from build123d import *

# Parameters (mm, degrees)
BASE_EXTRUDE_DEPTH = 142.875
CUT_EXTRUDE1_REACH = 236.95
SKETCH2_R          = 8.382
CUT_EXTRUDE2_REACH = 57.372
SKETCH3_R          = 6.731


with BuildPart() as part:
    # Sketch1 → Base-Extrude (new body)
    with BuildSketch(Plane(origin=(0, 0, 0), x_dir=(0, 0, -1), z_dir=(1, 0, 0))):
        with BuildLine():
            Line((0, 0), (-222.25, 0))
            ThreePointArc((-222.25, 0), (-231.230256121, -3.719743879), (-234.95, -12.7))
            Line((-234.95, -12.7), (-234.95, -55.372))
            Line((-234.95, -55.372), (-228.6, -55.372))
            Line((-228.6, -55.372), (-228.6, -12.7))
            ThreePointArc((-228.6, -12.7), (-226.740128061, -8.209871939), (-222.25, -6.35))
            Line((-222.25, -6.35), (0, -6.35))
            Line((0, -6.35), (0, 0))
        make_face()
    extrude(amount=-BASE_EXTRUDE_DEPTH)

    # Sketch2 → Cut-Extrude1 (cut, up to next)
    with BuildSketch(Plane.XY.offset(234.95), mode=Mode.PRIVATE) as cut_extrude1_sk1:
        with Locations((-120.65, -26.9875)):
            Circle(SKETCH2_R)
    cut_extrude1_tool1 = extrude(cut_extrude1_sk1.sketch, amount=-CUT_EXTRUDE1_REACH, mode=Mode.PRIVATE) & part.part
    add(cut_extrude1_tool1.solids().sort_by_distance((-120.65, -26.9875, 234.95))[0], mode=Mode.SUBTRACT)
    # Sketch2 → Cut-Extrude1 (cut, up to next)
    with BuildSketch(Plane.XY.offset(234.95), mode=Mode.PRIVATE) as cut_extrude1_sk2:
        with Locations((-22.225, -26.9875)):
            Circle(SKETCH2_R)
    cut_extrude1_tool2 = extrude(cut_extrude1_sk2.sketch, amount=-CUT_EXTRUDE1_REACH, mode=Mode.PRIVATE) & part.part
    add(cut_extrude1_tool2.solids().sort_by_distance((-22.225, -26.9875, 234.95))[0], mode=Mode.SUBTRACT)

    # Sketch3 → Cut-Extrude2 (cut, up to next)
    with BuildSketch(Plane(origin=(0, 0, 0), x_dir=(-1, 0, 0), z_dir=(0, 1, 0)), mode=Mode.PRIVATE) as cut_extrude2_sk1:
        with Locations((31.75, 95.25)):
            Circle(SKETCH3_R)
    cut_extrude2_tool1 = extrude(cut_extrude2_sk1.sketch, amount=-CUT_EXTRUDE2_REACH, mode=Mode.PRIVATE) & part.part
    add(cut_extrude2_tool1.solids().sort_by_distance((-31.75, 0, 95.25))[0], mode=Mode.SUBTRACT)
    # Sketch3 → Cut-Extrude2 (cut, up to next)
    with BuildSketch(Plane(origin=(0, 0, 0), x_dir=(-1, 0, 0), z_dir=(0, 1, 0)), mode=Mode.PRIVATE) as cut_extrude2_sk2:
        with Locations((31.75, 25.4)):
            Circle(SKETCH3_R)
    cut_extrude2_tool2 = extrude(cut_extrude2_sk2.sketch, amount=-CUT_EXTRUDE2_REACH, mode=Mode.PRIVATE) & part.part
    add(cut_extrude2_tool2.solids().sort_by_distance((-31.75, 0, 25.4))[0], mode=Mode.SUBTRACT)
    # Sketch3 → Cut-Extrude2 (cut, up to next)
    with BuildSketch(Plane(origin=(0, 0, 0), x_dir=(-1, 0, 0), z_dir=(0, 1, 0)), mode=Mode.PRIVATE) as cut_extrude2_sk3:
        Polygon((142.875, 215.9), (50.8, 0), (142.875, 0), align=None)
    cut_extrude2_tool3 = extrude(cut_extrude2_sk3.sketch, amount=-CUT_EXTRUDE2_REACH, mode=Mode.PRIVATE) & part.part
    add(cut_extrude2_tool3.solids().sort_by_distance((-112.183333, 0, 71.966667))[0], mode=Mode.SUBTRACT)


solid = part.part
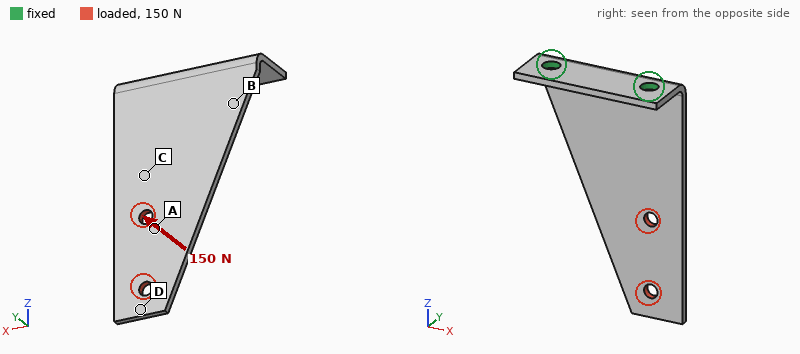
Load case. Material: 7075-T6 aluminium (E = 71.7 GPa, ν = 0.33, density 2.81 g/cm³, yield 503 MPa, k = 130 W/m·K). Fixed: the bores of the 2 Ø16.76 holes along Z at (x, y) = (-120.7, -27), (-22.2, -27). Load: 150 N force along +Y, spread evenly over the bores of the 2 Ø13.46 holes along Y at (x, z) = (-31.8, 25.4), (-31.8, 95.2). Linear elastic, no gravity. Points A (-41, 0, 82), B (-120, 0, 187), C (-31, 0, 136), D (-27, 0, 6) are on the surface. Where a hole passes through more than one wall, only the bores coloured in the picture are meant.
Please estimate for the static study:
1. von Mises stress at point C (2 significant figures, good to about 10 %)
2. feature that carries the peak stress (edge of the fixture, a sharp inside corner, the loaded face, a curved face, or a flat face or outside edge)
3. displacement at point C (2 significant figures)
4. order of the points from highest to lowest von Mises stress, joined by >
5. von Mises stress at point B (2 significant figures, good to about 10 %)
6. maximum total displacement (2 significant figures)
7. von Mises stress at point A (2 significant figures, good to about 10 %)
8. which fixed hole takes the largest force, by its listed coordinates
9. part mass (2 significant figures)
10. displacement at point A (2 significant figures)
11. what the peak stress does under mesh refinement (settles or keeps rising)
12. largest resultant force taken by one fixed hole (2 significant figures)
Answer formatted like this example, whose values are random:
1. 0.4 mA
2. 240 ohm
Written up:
1. 16 MPa
2. edge of the fixture
3. 0.69 mm
4. B > C > A > D
5. 22 MPa
6. 2.6 mm
7. 8.9 MPa
8. (-22.2, -27)
9. 520 g
10. 1.3 mm
11. keeps rising
12. 130 N
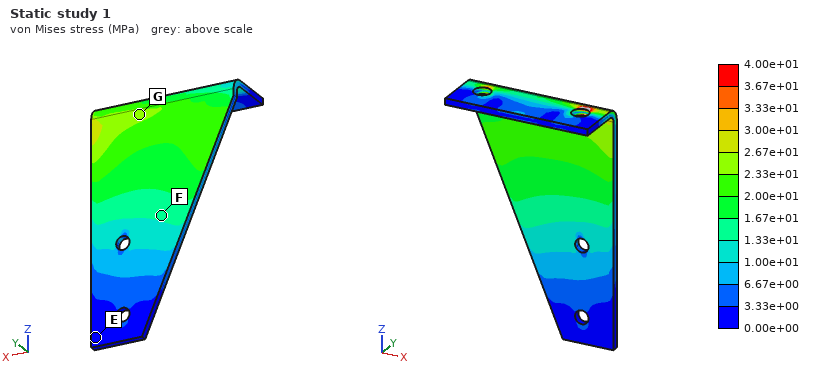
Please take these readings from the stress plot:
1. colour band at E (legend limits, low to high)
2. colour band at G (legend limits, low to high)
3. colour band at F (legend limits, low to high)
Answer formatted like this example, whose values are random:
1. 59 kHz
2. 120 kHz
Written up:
1. 0.00e+00 to 3.33e+00 MPa
2. 2.33e+01 to 2.67e+01 MPa
3. 1.33e+01 to 1.67e+01 MPa
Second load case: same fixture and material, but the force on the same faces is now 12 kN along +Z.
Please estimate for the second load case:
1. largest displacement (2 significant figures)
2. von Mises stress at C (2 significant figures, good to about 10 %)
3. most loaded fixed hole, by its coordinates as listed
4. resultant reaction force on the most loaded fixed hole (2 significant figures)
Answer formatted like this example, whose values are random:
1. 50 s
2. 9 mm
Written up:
1. 3.2 mm
2. 26 MPa
3. (-22.2, -27)
4. 11 kN
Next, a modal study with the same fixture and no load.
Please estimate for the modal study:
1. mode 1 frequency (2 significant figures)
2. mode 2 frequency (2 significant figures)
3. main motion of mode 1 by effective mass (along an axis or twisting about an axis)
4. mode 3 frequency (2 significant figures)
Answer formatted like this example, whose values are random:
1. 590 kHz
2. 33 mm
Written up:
1. 120 Hz
2. 570 Hz
3. along Y
4. 660 Hz
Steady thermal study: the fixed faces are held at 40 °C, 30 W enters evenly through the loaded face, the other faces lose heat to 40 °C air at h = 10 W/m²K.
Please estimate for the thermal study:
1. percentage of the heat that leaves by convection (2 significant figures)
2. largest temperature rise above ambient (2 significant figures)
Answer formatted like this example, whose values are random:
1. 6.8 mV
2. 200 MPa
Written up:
1. 40 %
2. 52 K
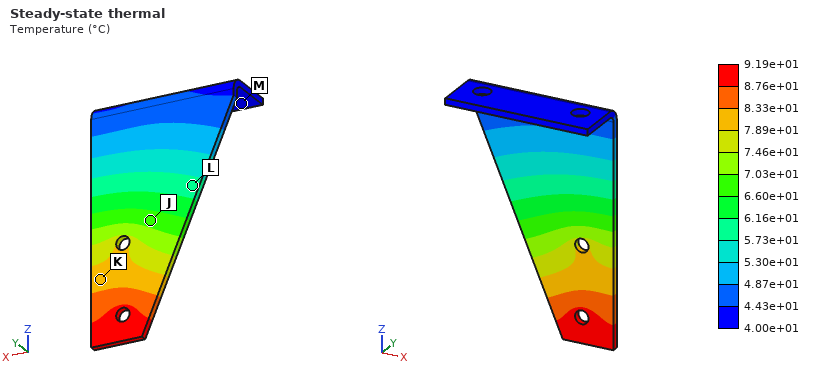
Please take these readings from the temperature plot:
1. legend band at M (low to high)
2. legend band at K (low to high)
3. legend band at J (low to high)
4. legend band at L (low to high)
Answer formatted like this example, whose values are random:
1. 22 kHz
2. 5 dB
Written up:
1. 4.00e+01 to 4.43e+01 °C
2. 7.89e+01 to 8.33e+01 °C
3. 6.60e+01 to 7.03e+01 °C
4. 5.73e+01 to 6.16e+01 °C
